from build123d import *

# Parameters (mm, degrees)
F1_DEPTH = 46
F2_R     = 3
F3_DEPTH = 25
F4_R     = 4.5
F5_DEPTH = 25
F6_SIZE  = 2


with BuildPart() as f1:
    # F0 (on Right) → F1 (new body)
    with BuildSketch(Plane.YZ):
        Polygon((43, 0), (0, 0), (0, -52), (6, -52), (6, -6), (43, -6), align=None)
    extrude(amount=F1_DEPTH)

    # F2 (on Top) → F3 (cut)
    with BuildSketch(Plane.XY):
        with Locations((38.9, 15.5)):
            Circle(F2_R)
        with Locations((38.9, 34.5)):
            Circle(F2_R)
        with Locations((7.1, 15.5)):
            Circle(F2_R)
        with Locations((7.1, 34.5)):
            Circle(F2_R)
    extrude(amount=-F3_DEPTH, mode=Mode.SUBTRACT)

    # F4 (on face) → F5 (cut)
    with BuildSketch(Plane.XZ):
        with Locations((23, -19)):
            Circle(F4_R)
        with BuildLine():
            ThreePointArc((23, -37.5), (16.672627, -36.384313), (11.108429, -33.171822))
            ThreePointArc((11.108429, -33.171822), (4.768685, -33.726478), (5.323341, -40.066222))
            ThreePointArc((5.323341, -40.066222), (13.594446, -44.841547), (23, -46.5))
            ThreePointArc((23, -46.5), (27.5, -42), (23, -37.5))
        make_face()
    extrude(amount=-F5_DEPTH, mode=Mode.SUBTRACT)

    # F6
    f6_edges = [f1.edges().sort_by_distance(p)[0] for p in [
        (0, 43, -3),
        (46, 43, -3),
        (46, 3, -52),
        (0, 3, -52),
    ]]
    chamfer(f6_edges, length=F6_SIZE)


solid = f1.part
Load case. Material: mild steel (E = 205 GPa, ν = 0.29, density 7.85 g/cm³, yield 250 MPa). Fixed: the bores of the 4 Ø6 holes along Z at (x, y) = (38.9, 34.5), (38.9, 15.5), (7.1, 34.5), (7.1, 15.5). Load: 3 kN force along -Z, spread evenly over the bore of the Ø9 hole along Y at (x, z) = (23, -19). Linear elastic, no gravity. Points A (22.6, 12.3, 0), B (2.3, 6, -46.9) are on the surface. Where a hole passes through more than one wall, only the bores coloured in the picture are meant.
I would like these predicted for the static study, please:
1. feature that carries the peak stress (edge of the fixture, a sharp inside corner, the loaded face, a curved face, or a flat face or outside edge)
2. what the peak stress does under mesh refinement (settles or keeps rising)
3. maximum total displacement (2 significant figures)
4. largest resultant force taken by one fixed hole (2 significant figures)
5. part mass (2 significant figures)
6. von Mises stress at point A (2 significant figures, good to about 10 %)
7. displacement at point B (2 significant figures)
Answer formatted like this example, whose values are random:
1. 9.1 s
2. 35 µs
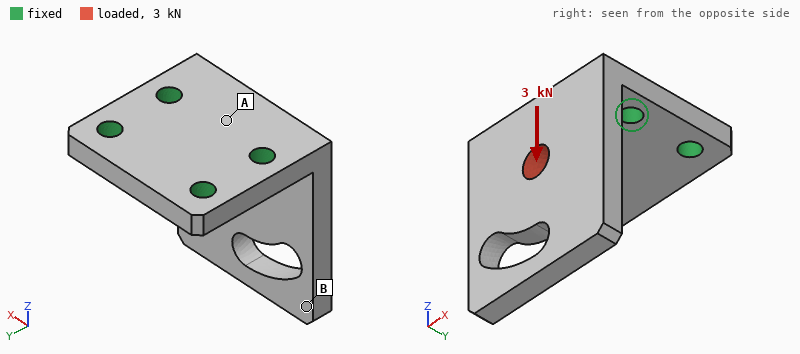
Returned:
1. edge of the fixture
2. keeps rising
3. 66 µm
4. 1.7 kN
5. 170 g
6. 43 MPa
7. 58 µm
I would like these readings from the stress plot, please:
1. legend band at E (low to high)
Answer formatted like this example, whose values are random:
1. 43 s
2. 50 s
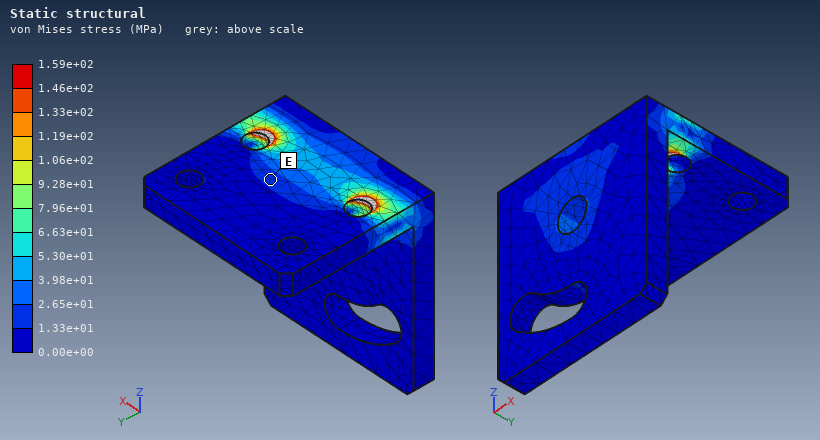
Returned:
1. 1.33e+01 to 2.65e+01 MPa
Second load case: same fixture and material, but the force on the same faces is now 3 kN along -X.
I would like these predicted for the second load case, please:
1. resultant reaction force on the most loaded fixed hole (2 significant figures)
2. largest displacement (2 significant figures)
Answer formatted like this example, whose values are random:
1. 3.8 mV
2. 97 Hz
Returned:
1. 2.2 kN
2. 31 µm
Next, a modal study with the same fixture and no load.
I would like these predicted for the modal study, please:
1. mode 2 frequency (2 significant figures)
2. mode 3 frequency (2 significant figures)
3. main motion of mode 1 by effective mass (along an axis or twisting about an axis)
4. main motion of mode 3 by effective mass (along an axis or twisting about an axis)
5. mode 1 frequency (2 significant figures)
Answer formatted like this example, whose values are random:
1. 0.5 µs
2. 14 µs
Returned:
1. 4100 Hz
2. 5500 Hz
3. along Y
4. along X
5. 1600 Hz
